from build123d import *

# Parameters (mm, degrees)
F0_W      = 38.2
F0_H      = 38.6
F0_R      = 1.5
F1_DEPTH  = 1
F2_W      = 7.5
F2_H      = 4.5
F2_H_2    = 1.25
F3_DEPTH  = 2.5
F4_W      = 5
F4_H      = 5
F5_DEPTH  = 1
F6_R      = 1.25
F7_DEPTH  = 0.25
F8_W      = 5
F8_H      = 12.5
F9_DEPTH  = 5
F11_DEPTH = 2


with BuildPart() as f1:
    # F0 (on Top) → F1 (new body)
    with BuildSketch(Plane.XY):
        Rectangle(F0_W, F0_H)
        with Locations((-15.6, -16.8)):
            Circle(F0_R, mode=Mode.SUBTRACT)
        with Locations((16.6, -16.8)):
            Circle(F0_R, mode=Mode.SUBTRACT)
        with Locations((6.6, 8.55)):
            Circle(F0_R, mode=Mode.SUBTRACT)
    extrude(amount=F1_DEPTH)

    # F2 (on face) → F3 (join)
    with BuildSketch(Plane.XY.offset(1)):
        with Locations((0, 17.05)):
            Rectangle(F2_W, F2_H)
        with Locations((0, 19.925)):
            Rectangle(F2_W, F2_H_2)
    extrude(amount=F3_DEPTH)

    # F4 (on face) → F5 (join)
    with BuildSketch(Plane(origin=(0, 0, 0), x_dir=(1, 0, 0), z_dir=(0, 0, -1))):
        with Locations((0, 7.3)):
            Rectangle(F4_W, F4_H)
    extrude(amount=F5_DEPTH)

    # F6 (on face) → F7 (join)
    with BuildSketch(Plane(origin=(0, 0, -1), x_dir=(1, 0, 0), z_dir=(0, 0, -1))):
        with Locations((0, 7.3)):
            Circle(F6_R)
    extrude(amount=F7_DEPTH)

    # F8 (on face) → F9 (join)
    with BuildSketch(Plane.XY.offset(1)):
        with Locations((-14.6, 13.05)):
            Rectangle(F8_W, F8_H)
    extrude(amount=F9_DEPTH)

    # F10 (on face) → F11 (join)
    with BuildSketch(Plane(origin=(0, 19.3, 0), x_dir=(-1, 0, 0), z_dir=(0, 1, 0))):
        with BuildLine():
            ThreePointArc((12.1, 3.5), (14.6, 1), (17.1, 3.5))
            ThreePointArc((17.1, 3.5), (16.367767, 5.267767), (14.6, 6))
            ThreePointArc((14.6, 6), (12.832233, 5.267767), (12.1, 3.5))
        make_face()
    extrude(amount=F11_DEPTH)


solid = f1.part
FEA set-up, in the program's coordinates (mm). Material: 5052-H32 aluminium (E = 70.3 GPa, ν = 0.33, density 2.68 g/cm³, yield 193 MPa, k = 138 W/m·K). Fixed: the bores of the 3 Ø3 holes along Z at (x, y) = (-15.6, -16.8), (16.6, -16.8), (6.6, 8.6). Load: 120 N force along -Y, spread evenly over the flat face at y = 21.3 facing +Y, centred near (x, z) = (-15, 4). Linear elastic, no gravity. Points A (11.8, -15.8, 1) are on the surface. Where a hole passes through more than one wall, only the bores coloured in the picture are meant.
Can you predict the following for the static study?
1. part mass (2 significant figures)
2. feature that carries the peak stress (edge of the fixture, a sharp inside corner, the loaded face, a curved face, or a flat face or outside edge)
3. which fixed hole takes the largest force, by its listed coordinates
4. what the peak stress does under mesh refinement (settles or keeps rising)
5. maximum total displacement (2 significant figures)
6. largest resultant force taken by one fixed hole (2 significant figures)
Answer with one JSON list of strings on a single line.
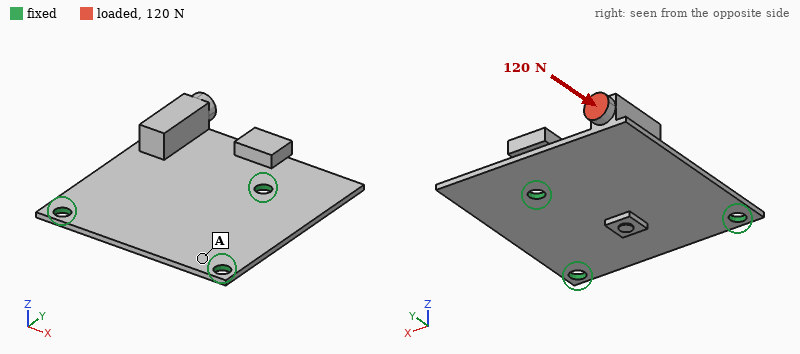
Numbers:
["5.2 g", "edge of the fixture", "(-15.6, -16.8)", "keeps rising", "0.32 mm", "77 N"]
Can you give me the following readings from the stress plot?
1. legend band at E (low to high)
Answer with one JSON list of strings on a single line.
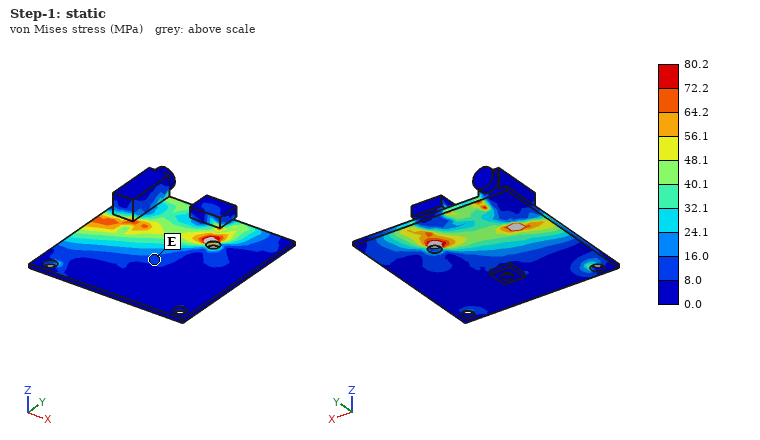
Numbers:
["8.0 to 16.0 MPa"]
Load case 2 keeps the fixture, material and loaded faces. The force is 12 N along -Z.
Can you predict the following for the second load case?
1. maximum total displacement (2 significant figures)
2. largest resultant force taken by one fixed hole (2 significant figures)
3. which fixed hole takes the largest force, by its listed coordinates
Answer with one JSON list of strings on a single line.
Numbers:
["0.29 mm", "13 N", "(6.6, 8.6)"]
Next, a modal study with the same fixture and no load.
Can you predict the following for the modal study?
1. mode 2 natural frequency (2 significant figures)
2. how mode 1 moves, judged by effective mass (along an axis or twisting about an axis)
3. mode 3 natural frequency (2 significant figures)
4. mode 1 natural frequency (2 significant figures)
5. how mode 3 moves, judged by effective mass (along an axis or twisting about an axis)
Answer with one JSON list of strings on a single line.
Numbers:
["3700 Hz", "along Z", "5100 Hz", "1200 Hz", "along Z"]
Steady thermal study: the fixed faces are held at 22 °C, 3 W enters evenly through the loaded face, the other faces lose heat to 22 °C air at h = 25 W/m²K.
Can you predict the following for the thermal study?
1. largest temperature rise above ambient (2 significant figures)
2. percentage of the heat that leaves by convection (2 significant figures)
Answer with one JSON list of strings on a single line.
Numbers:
["22 K", "14 %"]
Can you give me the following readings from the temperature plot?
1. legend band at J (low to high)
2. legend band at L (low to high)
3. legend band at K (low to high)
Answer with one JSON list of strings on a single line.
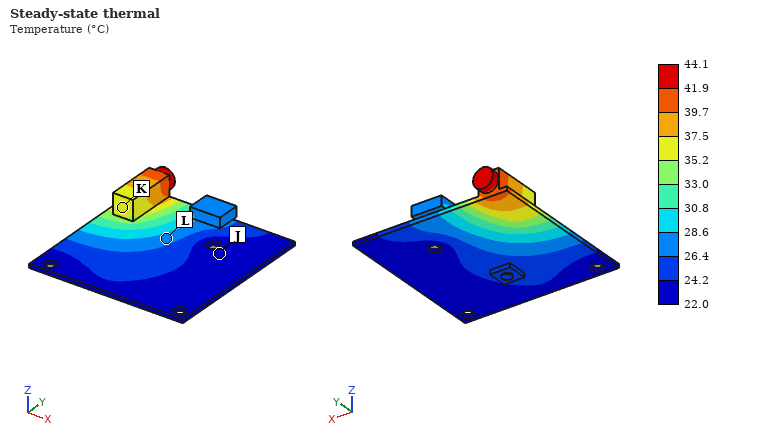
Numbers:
["22.0 to 24.2 °C", "26.4 to 28.6 °C", "35.2 to 37.5 °C"]
